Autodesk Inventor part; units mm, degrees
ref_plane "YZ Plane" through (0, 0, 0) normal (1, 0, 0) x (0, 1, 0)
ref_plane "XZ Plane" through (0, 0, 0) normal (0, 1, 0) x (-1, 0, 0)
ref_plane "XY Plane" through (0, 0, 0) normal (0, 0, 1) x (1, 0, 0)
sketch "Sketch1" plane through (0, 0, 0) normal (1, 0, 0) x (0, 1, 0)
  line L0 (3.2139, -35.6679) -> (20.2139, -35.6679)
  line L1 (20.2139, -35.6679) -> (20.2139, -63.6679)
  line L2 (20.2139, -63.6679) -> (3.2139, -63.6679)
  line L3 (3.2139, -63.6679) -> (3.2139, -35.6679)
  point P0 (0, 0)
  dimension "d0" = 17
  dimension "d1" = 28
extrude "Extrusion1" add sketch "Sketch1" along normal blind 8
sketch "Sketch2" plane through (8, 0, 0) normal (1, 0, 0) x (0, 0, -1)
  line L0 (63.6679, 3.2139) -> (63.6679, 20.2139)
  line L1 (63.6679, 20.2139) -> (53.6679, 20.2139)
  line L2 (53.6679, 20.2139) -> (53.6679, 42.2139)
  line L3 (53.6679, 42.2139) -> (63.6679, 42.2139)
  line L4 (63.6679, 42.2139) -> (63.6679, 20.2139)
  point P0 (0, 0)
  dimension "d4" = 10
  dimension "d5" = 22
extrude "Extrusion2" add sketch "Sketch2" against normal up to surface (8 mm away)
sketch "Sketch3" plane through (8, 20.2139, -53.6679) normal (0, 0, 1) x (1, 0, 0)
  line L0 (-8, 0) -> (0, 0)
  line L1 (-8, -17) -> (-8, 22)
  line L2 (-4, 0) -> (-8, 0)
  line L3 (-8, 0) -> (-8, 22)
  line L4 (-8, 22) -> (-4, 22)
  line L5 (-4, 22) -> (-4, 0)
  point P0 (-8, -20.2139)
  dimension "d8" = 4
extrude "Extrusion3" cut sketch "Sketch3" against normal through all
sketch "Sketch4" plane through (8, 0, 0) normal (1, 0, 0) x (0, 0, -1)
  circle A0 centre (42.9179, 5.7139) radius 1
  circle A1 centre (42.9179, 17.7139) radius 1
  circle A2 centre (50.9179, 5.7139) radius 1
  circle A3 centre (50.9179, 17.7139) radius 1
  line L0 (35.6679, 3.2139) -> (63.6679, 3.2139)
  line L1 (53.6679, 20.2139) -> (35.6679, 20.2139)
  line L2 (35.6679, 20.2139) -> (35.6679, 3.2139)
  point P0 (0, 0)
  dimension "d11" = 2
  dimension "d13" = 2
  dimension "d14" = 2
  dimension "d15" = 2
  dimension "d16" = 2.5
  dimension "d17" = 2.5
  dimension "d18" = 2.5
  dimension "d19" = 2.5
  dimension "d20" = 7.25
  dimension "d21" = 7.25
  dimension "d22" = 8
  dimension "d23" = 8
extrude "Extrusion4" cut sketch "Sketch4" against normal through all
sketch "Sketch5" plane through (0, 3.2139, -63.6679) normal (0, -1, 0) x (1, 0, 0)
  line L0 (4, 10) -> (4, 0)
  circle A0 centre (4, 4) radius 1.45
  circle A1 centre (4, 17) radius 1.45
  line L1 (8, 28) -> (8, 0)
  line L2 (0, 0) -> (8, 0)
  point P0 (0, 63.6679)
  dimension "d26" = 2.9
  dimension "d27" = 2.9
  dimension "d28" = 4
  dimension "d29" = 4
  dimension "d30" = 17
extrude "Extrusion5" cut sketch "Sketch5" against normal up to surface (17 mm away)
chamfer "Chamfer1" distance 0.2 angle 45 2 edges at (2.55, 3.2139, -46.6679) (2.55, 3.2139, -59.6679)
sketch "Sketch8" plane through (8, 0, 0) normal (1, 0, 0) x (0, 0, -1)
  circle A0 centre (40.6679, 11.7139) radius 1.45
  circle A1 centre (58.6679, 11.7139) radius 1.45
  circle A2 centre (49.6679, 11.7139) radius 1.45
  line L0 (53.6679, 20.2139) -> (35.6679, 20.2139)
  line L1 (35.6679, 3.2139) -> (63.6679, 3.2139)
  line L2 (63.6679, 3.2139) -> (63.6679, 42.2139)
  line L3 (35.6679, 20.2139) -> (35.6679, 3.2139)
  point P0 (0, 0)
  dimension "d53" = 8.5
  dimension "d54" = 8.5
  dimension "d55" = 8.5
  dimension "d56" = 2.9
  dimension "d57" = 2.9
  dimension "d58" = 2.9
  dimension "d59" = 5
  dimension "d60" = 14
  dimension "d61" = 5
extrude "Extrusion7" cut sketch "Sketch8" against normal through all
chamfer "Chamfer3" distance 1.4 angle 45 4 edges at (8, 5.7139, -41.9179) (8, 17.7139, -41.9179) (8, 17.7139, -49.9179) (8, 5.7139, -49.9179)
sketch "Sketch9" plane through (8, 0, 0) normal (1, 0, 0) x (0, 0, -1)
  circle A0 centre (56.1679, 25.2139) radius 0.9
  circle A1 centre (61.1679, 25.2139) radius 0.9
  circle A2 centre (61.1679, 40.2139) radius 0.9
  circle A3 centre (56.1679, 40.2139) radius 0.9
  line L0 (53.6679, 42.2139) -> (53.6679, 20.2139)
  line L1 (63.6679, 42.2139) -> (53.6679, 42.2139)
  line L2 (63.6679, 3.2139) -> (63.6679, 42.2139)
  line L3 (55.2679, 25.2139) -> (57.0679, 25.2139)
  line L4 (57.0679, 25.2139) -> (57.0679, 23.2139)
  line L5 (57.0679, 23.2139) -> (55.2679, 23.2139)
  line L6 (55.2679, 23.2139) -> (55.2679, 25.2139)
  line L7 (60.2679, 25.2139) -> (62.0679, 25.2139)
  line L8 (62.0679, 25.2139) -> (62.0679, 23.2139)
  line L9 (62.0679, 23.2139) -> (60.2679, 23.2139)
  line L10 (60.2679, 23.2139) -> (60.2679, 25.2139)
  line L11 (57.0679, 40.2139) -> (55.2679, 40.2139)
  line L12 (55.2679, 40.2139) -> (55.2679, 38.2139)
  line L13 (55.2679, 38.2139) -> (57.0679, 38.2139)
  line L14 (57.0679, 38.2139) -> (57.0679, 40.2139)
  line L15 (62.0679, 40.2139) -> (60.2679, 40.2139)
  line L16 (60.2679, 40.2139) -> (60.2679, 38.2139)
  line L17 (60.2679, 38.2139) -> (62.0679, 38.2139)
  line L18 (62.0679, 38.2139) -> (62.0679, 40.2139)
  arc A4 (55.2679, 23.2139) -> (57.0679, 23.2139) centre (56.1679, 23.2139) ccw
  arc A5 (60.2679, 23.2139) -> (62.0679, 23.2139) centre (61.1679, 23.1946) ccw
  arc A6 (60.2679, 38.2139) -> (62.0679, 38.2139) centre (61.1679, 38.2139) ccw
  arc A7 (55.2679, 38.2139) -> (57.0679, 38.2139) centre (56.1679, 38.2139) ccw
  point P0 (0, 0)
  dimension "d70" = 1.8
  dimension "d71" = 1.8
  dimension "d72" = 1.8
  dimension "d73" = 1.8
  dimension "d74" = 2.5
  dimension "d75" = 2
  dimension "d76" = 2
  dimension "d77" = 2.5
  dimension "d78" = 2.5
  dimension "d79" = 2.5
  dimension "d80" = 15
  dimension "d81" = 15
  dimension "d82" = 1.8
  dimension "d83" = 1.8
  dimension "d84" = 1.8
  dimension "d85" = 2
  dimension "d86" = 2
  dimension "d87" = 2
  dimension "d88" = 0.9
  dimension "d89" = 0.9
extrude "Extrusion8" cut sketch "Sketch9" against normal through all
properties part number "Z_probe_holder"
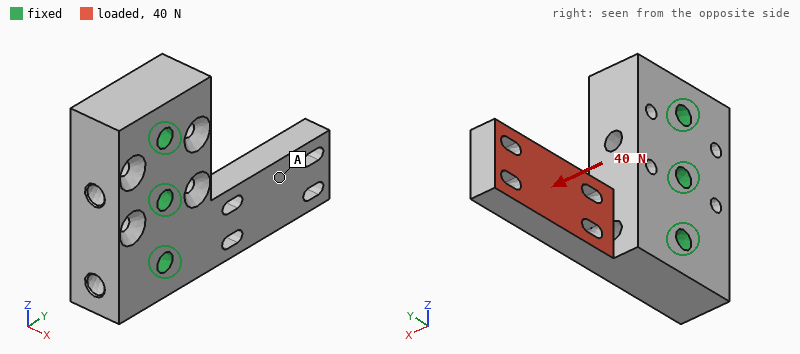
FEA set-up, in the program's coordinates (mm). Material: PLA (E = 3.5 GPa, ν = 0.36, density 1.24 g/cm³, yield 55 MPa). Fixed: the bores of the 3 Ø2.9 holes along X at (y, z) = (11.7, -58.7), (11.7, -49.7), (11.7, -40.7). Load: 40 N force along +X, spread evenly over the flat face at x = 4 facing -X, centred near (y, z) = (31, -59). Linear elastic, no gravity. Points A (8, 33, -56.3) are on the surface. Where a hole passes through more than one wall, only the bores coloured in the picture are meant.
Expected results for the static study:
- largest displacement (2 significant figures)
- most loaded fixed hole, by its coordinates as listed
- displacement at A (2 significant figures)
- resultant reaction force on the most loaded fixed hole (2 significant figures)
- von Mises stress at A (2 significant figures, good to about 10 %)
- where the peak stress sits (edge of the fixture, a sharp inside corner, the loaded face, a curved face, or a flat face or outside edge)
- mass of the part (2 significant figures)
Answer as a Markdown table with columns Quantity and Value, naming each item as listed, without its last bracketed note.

| Quantity | Value |
|---|---|
| largest displacement | 0.56 mm |
| most loaded fixed hole, by its coordinates as listed | (11.7, -58.7) |
| displacement at A | 0.29 mm |
| resultant reaction force on the most loaded fixed hole | 28 N |
| von Mises stress at A | 2.8 MPa |
| where the peak stress sits | the loaded face |
| mass of the part | 5.1 g |
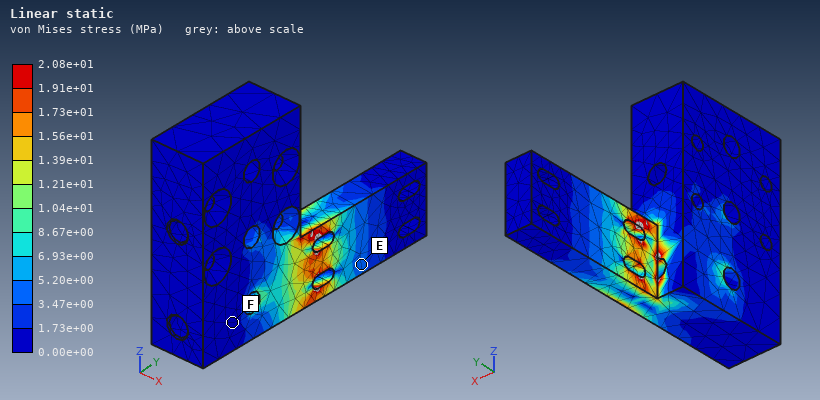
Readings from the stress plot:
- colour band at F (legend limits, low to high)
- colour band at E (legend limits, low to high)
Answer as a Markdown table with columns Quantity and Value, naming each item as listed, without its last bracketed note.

| Quantity | Value |
|---|---|
| colour band at F | 0.00e+00 to 1.73e+00 MPa |
| colour band at E | 3.47e+00 to 5.20e+00 MPa |
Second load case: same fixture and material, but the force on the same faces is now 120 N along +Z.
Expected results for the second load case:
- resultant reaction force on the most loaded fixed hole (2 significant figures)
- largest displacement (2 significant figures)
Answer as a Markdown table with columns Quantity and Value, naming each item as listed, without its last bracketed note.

| Quantity | Value |
|---|---|
| resultant reaction force on the most loaded fixed hole | 180 N |
| largest displacement | 0.44 mm |
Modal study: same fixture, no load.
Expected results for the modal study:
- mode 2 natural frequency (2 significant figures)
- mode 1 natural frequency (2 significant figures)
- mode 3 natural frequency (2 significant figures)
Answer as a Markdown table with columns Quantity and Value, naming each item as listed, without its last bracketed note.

| Quantity | Value |
|---|---|
| mode 2 natural frequency | 3500 Hz |
| mode 1 natural frequency | 1700 Hz |
| mode 3 natural frequency | 6600 Hz |
